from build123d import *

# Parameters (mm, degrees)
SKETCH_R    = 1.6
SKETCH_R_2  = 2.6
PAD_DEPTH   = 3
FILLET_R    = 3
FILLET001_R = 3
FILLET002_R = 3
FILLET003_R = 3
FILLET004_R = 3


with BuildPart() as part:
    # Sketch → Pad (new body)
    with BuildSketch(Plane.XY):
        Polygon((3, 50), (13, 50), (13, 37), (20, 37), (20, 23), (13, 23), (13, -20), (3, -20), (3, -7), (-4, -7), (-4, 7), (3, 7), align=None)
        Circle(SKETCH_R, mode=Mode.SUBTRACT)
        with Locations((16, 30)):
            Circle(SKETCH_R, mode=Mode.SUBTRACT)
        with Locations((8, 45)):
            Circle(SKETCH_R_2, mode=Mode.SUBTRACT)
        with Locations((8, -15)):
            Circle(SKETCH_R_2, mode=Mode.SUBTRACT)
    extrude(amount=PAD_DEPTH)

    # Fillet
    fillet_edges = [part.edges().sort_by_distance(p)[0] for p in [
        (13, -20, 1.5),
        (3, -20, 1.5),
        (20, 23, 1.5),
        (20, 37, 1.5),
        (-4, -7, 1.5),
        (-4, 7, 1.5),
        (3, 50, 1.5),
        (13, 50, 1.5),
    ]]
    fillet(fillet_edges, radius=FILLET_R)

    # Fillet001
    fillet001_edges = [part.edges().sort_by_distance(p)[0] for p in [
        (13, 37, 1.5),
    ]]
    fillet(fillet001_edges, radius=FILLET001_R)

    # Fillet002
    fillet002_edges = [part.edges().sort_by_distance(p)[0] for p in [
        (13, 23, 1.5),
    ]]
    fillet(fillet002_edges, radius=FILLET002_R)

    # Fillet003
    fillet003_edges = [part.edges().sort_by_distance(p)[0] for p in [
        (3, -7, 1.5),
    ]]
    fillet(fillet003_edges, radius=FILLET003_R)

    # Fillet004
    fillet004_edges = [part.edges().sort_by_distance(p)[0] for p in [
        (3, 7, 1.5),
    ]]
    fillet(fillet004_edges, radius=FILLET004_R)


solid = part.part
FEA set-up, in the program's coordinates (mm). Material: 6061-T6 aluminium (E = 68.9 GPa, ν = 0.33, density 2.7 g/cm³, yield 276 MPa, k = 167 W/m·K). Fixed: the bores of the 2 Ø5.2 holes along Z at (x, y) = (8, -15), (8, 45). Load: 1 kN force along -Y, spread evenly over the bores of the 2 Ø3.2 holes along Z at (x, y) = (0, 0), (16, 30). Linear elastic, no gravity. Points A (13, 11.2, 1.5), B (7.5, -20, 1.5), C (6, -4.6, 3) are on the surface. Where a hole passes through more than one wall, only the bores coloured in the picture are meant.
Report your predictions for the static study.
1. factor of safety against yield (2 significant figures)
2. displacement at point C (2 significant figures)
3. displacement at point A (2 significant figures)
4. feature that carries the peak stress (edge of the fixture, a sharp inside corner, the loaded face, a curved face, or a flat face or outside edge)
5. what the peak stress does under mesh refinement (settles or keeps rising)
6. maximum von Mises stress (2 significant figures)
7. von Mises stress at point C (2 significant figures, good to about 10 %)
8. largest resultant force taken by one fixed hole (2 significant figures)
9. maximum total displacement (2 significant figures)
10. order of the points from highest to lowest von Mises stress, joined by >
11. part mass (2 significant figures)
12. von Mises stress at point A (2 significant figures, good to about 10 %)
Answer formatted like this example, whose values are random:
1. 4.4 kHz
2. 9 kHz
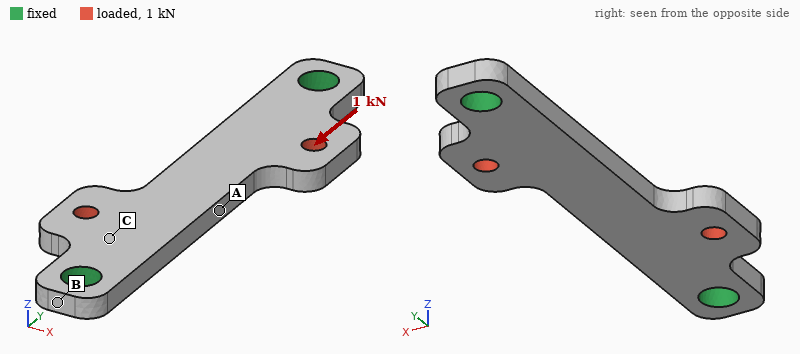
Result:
1. 3.4
2. 8.3 µm
3. 24 µm
4. a curved face
5. settles
6. 81 MPa
7. 20 MPa
8. 500 N
9. 27 µm
10. A > C > B
11. 6.7 g
12. 38 MPa
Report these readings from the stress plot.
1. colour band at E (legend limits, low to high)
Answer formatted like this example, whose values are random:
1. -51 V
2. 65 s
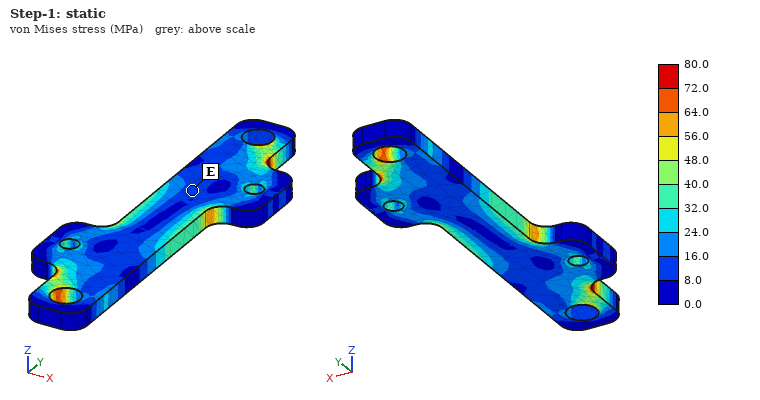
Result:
1. 8.0 to 16.0 MPa
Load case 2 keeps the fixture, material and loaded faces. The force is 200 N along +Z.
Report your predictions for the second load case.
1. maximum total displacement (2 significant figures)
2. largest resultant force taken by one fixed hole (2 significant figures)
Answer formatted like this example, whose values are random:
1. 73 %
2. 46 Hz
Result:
1. 68 µm
2. 100 N
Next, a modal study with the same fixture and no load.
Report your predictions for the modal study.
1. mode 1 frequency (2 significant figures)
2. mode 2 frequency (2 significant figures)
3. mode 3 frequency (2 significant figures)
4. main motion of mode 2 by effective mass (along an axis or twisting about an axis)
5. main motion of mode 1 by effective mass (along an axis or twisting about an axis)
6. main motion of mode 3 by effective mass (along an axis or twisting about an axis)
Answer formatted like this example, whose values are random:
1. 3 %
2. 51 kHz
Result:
1. 4400 Hz
2. 7900 Hz
3. 11 kHz
4. twisting about Y
5. along Z
6. along X
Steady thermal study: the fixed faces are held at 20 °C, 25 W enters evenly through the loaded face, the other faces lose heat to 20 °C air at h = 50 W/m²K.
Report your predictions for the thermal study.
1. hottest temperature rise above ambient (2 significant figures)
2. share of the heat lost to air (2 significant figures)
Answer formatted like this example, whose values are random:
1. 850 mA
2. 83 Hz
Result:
1. 37 K
2. 8.6 %
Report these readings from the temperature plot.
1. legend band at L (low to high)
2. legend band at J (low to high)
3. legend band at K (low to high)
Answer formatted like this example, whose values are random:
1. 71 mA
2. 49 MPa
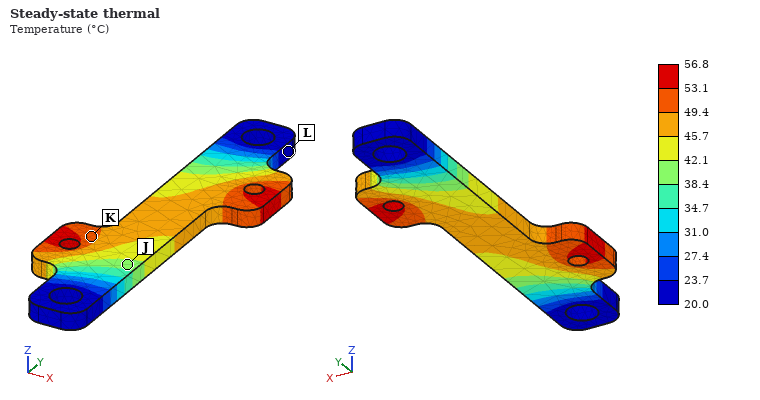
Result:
1. 20.0 to 23.7 °C
2. 38.4 to 42.1 °C
3. 49.4 to 53.1 °C
